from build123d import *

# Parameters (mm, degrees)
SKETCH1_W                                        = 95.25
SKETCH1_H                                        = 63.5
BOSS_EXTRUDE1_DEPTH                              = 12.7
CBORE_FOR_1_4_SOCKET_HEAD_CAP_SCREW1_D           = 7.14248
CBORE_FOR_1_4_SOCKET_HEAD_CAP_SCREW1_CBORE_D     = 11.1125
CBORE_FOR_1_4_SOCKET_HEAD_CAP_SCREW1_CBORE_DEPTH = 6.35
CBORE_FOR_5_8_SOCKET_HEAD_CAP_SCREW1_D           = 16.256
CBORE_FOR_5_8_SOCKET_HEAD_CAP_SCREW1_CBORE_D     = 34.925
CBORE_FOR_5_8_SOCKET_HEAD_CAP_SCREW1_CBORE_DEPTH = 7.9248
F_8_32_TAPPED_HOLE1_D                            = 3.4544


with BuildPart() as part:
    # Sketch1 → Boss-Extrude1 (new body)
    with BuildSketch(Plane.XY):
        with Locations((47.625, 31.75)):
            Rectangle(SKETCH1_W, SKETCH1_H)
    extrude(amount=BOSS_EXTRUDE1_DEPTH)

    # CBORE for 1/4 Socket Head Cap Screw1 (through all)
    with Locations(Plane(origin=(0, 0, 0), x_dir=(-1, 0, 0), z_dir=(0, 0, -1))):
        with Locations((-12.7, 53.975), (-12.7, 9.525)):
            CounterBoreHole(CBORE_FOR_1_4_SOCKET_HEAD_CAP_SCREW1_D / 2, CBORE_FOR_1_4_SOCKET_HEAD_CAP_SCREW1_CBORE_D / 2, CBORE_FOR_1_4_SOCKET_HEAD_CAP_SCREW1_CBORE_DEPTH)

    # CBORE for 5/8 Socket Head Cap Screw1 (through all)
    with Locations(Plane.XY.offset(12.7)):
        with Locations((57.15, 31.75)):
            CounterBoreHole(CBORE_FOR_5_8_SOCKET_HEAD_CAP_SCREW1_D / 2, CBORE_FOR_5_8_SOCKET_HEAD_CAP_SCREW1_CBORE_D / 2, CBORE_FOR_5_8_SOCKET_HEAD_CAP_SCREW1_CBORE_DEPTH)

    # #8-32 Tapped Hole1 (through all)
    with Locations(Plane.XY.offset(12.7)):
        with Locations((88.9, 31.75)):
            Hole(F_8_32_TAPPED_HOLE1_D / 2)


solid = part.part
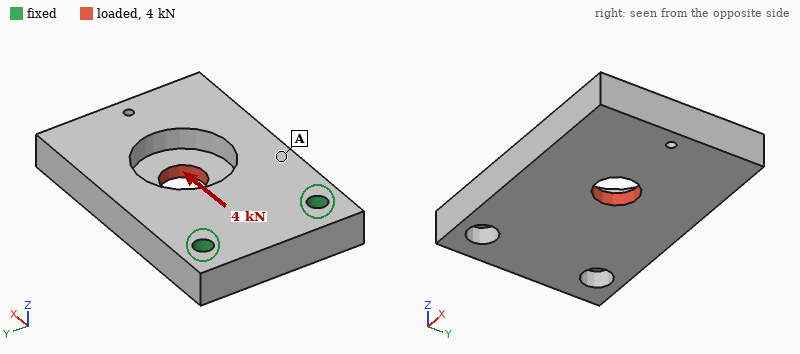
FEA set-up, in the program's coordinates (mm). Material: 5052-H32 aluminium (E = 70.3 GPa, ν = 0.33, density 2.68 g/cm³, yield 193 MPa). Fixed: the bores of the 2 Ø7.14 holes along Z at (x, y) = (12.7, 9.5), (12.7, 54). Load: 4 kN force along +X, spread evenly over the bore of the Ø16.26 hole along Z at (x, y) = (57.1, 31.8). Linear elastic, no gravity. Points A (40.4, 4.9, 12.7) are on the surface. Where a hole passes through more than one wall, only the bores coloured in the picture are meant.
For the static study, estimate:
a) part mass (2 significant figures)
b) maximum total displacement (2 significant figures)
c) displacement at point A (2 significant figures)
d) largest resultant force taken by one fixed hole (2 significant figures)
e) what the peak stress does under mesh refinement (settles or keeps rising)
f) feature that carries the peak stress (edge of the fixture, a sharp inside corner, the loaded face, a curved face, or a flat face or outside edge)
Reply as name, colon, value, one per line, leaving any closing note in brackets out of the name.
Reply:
part mass: 180 g
maximum total displacement: 0.12 mm
displacement at point A: 0.029 mm
largest resultant force taken by one fixed hole: 2.0 kN
what the peak stress does under mesh refinement: keeps rising
feature that carries the peak stress: edge of the fixture
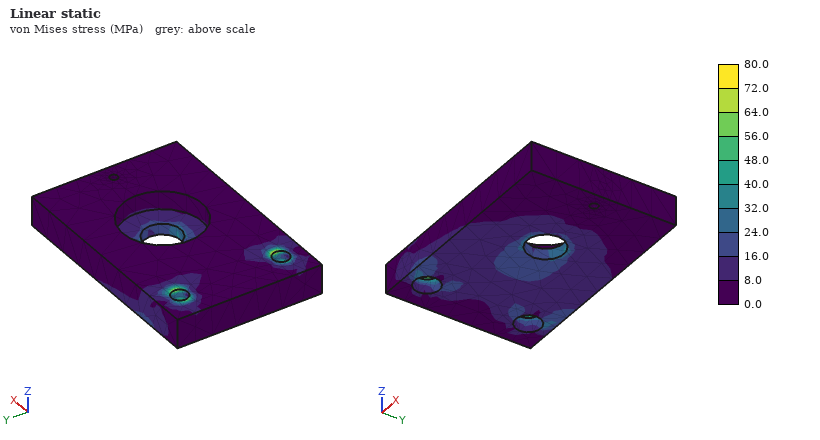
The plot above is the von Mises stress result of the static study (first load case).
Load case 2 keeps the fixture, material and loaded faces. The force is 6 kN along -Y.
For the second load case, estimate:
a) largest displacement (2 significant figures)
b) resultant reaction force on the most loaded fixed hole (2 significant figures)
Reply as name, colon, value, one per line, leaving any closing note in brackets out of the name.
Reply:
largest displacement: 62 µm
resultant reaction force on the most loaded fixed hole: 6.4 kN
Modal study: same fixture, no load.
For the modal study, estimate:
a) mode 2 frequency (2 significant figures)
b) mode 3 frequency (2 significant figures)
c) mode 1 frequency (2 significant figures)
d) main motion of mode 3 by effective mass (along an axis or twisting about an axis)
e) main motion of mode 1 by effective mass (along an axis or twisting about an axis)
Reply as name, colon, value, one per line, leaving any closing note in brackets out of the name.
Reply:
mode 2 frequency: 3300 Hz
mode 3 frequency: 4800 Hz
mode 1 frequency: 1100 Hz
main motion of mode 3 by effective mass: along Y
main motion of mode 1 by effective mass: along Z
